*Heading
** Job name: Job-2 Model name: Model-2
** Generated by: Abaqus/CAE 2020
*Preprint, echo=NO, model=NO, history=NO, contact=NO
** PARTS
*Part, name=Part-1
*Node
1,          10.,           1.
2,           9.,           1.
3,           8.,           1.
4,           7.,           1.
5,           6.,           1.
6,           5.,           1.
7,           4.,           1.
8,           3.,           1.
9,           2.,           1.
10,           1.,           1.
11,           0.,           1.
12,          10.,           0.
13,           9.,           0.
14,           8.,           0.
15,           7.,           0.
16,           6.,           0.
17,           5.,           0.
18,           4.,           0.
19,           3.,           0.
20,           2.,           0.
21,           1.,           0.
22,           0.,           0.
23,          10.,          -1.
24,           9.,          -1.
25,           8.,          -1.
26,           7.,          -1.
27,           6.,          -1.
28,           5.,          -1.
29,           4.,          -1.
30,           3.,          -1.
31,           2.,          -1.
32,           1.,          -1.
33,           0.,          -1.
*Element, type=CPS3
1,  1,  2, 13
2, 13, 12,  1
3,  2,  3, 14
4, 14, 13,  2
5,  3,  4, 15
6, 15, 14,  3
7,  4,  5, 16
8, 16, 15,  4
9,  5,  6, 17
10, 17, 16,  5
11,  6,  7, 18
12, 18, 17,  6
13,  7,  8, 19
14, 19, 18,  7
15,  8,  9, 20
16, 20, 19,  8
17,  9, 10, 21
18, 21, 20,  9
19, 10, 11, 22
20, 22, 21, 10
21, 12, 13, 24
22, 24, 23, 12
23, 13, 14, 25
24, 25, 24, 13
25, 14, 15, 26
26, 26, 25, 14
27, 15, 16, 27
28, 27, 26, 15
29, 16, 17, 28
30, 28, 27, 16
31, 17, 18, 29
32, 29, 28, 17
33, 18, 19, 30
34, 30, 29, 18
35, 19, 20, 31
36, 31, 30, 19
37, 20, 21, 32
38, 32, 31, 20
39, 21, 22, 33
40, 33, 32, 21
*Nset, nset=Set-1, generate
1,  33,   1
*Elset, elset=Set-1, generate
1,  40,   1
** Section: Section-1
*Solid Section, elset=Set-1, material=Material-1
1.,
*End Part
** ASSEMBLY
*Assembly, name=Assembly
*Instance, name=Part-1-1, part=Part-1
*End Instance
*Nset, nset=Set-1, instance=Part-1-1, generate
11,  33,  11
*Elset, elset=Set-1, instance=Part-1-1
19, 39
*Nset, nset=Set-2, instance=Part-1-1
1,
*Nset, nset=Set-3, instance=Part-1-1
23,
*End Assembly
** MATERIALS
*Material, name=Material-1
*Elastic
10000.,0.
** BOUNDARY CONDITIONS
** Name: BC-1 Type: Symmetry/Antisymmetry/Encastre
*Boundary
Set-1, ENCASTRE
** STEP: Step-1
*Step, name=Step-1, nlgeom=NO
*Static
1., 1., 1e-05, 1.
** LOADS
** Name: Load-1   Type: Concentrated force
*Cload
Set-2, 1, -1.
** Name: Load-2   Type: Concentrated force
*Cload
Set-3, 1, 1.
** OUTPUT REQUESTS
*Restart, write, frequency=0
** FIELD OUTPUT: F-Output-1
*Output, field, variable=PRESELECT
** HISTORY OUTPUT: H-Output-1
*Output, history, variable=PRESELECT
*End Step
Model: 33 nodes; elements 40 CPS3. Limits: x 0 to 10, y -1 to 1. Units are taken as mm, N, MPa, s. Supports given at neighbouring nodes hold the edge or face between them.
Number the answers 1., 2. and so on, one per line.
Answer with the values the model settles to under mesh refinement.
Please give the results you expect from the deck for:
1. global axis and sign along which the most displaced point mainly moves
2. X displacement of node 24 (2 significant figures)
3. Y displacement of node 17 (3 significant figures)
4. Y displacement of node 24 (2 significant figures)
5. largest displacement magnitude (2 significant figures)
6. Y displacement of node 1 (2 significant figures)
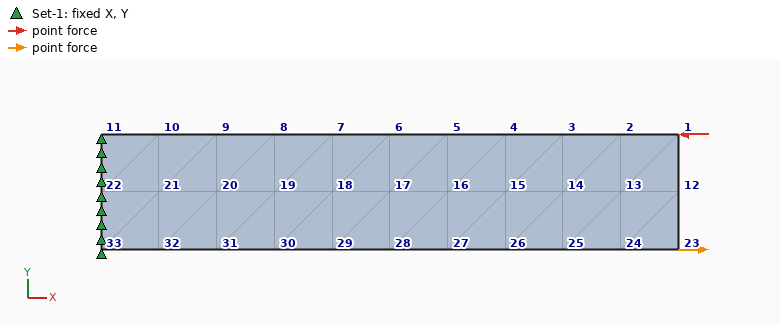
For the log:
1. +Y
2. 0.0027 mm
3. 0.00375 mm
4. 0.012 mm
5. 0.016 mm
6. 0.015 mm
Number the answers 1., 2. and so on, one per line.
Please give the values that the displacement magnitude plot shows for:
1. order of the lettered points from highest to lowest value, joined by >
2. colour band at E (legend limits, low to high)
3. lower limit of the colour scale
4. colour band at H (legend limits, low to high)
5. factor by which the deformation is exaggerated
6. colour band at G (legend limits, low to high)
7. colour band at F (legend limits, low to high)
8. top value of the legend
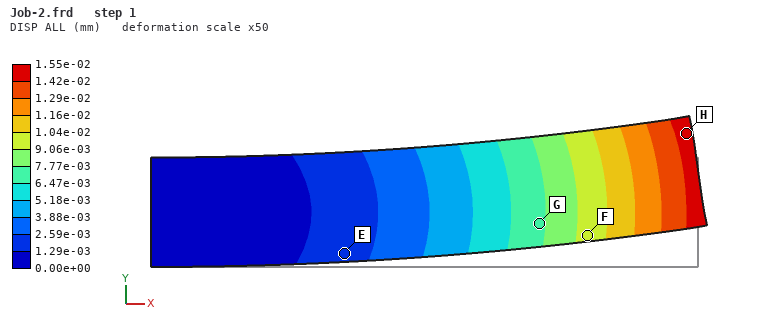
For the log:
1. H > F > G > E
2. 1.29e-03 to 2.59e-03 mm
3. 0.00e+00 mm
4. 1.42e-02 to 1.55e-02 mm
5. 50
6. 6.47e-03 to 7.77e-03 mm
7. 9.06e-03 to 1.04e-02 mm
8. 1.55e-02 mm
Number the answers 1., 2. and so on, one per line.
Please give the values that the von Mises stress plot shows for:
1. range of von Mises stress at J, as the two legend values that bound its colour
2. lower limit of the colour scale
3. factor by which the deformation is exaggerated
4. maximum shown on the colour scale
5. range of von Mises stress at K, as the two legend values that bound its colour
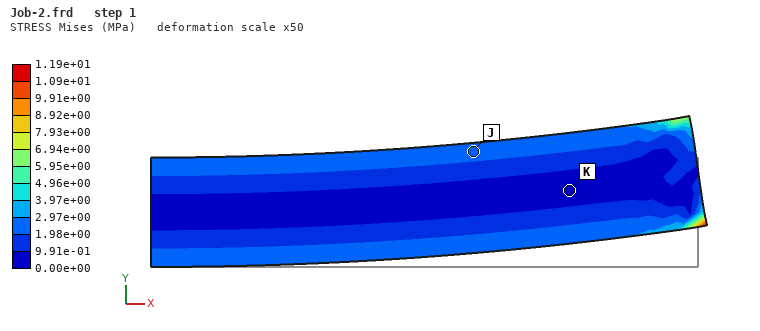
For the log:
1. 1.98e+00 to 2.97e+00 MPa
2. 0.00e+00 MPa
3. 50
4. 1.19e+01 MPa
5. 0.00e+00 to 9.91e-01 MPa
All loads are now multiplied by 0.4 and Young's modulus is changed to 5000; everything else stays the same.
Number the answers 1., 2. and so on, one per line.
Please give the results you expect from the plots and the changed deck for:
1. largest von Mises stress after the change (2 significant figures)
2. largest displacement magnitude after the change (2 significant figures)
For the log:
1. 4.8 MPa
2. 0.012 mm
